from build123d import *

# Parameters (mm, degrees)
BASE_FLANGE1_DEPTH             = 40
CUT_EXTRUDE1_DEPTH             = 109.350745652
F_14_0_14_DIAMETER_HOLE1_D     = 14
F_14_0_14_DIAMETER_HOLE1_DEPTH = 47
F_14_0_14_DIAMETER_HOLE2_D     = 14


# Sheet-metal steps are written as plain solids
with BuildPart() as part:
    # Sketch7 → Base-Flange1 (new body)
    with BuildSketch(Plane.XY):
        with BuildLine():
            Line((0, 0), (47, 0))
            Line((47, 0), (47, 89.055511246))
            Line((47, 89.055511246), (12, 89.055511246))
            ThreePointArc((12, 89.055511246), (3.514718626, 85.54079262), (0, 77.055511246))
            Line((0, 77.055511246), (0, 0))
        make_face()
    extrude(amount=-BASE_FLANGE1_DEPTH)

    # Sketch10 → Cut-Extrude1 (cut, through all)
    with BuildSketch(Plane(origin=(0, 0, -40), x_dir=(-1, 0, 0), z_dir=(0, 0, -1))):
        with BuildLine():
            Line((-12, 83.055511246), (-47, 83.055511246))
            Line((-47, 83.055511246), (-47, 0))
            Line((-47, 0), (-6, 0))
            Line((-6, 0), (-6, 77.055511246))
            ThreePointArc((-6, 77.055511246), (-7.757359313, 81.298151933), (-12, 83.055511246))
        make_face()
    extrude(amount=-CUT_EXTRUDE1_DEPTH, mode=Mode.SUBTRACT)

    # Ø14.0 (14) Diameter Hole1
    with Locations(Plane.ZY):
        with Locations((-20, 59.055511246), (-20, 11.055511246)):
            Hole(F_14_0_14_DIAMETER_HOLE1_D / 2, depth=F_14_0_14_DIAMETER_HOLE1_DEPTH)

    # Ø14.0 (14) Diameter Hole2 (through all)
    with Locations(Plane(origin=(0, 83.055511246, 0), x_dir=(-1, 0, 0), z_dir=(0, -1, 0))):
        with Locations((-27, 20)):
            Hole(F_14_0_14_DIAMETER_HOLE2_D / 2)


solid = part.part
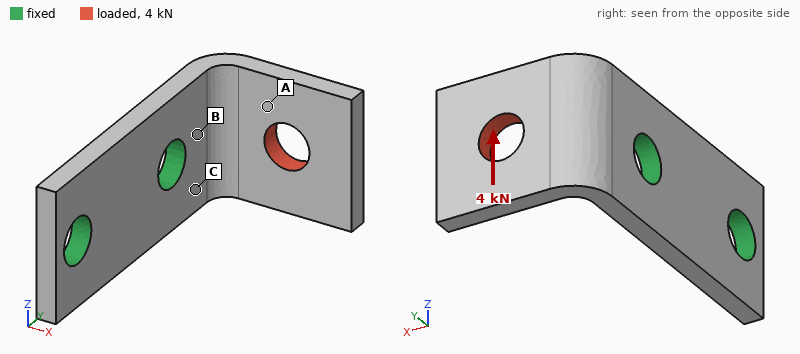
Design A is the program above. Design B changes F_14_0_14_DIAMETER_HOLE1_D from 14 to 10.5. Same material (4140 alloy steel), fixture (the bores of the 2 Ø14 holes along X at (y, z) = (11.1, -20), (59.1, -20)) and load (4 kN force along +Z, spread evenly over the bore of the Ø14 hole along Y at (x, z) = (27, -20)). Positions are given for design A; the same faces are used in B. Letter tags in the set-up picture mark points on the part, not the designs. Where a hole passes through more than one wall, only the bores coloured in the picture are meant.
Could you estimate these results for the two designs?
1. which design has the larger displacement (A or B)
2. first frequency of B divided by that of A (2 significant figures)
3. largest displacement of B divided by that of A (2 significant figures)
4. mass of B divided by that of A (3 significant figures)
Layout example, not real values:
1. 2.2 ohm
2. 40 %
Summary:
1. B
2. 0.95
3. 1.2
4. 1.03
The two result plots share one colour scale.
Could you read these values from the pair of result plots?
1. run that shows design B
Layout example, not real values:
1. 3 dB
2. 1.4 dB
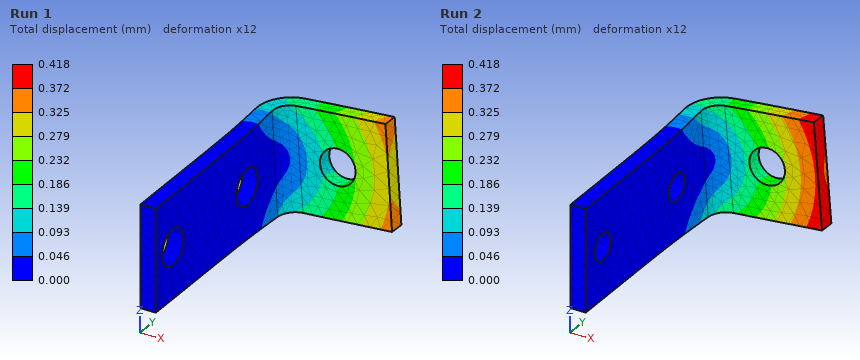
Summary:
1. Run 2
